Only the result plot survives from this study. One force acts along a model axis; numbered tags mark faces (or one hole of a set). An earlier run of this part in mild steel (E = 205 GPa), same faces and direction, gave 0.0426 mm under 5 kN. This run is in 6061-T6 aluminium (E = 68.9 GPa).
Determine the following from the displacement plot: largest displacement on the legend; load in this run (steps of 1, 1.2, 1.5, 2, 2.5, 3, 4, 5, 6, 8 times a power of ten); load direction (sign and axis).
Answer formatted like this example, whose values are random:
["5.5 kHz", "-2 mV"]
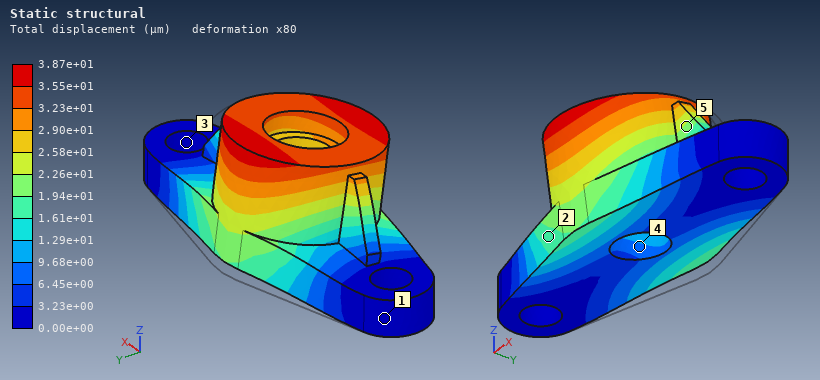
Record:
["3.87e+01 µm", "1.5 kN", "-Y"]
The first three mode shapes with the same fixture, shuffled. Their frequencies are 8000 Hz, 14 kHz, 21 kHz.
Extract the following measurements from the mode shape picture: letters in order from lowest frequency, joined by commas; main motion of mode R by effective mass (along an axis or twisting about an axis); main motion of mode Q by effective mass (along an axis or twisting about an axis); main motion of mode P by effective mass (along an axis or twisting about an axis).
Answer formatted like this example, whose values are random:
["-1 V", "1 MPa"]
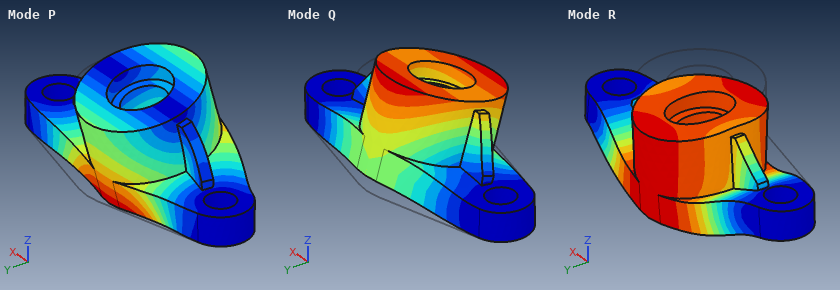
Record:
["Q, R, P", "along Z", "along Y", "along Y"]
